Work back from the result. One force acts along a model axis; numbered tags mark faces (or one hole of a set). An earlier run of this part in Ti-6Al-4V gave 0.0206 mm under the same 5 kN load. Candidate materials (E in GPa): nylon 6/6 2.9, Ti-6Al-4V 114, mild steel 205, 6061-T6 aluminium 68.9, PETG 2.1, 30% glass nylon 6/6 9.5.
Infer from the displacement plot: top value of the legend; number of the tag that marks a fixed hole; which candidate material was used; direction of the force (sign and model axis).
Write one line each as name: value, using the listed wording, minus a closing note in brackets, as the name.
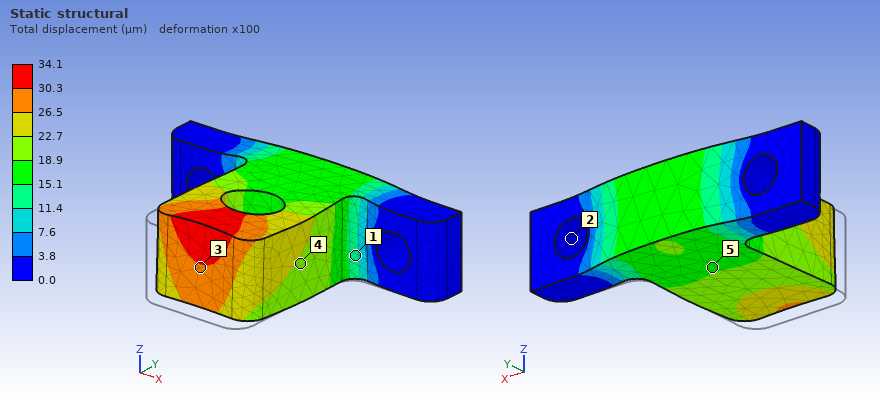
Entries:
top value of the legend: 34.1 µm
number of the tag that marks a fixed hole: 2
which candidate material was used: 6061-T6 aluminium
direction of the force: +Y
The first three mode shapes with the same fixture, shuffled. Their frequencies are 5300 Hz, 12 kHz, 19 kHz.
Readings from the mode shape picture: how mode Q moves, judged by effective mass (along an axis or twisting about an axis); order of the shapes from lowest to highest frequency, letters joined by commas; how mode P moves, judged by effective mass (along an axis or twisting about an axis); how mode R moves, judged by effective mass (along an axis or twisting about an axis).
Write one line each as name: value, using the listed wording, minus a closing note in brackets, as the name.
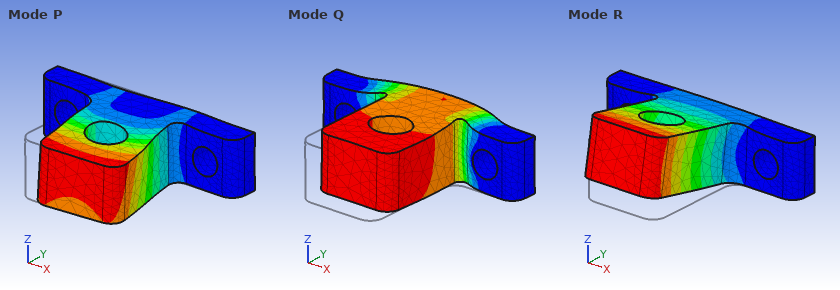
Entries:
how mode Q moves, judged by effective mass: along Y
order of the shapes from lowest to highest frequency, letters joined by commas: R, P, Q
how mode P moves, judged by effective mass: along X
how mode R moves, judged by effective mass: along Z
